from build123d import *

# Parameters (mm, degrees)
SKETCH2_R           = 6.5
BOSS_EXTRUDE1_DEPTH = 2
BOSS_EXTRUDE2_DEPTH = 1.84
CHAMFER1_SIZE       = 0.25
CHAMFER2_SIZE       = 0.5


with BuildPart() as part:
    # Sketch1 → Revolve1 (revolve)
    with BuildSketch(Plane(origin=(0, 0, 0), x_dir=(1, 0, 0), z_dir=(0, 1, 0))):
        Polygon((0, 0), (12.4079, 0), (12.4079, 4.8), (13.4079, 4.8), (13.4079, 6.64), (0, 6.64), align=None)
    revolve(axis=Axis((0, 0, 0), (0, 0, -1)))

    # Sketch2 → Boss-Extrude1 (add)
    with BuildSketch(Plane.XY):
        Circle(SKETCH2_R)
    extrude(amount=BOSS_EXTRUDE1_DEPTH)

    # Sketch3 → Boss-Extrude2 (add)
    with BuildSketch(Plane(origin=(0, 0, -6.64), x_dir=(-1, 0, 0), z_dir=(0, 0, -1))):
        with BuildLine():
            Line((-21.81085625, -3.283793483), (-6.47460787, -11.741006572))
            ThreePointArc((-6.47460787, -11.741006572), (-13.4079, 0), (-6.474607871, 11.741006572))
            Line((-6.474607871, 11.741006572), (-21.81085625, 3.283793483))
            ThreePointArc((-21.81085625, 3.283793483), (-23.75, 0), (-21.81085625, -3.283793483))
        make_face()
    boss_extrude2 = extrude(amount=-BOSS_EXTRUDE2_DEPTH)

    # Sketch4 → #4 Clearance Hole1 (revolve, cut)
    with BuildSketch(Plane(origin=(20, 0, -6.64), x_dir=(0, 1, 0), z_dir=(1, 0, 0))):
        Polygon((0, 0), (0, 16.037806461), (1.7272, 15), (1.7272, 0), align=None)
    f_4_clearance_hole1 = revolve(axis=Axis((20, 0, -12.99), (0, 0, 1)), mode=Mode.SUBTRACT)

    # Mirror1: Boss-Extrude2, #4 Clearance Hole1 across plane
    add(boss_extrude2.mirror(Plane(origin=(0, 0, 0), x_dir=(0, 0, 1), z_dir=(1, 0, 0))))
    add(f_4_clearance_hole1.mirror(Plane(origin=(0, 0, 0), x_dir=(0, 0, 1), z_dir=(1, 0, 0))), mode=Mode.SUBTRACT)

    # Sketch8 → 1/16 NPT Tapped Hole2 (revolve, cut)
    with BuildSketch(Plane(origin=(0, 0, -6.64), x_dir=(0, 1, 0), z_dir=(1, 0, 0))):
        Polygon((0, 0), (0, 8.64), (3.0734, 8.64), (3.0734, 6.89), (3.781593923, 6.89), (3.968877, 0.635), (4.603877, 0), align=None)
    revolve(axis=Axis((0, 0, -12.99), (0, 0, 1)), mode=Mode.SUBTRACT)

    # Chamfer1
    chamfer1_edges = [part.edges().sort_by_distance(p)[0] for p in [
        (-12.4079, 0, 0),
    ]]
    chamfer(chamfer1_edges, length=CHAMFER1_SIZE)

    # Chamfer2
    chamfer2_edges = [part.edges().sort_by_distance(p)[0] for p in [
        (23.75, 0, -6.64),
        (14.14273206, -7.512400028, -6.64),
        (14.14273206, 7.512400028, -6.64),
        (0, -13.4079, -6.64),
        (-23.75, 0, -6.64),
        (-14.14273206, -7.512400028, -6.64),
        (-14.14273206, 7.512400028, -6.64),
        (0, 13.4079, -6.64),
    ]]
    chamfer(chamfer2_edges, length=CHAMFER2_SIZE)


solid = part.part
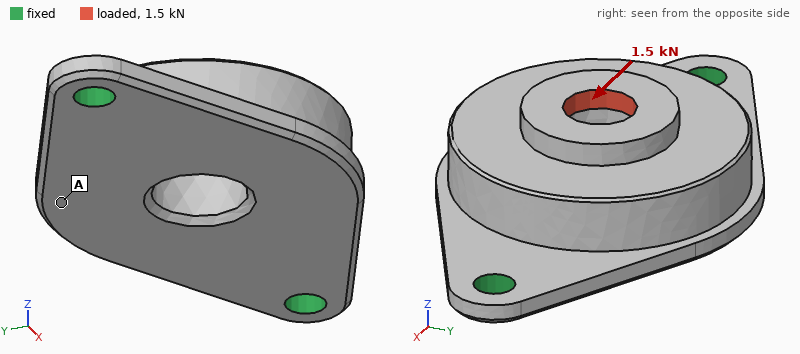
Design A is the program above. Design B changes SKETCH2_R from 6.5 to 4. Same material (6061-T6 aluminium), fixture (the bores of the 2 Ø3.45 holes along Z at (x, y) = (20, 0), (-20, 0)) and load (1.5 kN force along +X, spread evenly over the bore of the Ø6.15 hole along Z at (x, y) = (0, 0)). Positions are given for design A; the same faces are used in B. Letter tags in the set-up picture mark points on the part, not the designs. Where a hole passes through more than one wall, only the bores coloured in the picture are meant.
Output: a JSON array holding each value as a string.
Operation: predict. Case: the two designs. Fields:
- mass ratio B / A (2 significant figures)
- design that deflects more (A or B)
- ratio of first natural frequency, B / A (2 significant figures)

["0.95", "B", "1.0"]
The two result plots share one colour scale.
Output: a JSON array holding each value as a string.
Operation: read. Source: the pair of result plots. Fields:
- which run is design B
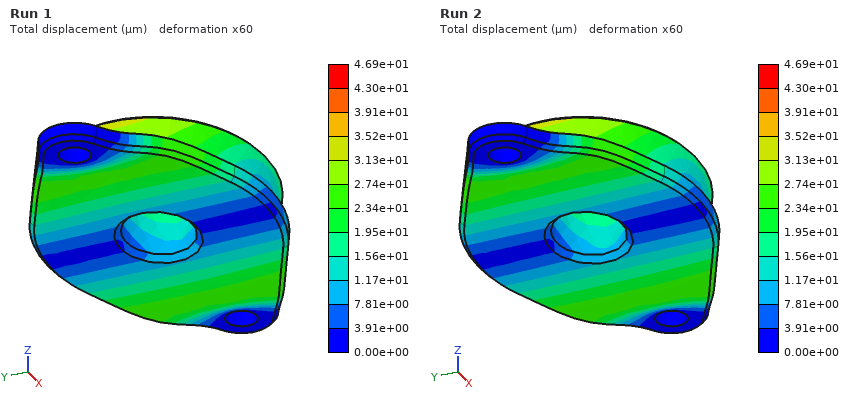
["Run 2"]
